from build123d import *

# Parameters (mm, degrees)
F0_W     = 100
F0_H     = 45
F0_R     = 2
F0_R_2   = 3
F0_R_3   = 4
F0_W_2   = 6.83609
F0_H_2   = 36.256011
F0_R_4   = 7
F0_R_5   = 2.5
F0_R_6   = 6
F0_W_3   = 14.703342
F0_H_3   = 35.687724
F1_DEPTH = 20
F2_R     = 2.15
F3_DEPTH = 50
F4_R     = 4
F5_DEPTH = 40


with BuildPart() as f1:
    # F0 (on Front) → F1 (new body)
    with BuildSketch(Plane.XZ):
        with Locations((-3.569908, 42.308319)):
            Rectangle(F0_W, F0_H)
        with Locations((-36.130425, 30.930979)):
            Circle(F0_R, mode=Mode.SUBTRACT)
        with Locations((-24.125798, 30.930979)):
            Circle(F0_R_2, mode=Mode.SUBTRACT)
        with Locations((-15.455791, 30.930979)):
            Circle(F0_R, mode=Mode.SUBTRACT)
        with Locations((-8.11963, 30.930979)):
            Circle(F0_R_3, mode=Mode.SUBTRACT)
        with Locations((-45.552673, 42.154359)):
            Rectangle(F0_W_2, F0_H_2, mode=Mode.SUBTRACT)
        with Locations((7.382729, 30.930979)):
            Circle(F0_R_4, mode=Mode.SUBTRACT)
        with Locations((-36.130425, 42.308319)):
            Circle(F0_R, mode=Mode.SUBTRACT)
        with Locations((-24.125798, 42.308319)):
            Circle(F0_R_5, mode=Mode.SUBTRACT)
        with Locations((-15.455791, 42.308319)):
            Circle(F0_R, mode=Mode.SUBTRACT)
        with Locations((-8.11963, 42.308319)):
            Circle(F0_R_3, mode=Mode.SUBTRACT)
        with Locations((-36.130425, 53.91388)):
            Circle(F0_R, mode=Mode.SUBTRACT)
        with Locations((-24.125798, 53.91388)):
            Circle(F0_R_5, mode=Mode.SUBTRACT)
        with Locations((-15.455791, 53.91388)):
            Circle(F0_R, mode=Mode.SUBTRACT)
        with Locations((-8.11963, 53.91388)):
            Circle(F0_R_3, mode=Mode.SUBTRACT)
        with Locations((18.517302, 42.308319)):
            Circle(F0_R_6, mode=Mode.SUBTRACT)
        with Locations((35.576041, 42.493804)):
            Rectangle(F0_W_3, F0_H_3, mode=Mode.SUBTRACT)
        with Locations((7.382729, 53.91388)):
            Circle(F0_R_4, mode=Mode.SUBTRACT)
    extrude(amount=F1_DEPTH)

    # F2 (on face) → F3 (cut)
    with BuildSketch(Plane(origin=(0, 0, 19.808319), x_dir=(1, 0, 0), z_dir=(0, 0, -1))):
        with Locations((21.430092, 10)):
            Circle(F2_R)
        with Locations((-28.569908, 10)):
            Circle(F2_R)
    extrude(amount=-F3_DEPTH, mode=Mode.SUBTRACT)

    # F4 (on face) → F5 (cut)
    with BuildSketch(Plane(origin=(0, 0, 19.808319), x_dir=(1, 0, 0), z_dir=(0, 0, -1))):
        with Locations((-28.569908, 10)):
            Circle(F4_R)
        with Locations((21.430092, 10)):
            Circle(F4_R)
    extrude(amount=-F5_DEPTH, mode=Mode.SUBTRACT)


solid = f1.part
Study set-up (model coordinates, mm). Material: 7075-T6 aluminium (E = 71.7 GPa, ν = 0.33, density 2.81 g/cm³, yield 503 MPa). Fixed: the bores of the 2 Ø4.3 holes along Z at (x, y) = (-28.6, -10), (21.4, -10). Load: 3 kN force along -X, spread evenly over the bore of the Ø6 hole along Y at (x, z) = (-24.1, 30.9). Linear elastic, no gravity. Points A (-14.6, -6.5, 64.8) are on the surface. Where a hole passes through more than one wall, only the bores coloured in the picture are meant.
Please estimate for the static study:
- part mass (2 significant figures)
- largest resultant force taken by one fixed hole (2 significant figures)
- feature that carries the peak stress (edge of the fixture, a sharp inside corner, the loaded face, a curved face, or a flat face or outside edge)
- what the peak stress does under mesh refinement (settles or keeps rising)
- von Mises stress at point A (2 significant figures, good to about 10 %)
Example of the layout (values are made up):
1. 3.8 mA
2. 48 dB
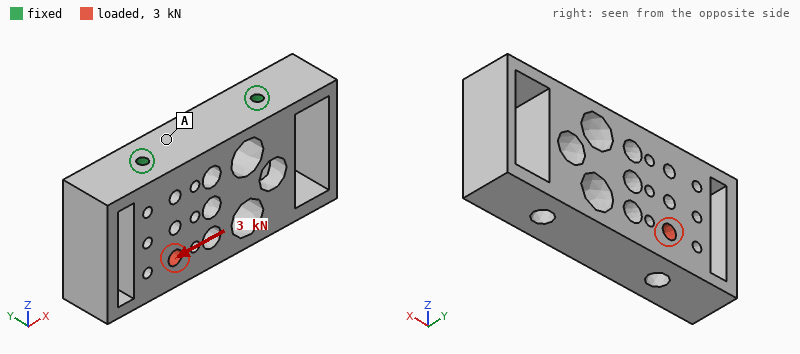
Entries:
1. 160 g
2. 2.4 kN
3. edge of the fixture
4. keeps rising
5. 7.4 MPa
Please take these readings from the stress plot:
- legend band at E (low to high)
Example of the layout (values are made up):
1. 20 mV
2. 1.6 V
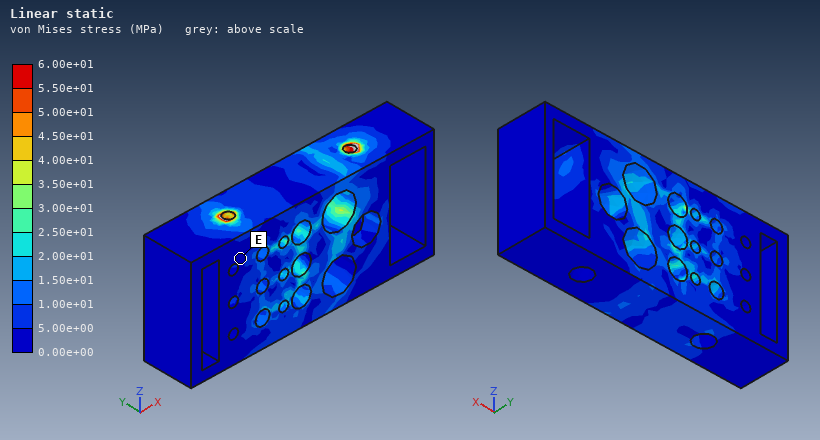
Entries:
1. 0.00e+00 to 5.00e+00 MPa
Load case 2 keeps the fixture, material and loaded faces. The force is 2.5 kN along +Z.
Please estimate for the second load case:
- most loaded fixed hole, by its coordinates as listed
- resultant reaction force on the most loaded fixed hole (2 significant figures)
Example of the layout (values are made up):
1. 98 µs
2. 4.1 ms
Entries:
1. (-28.6, -10)
2. 2.2 kN
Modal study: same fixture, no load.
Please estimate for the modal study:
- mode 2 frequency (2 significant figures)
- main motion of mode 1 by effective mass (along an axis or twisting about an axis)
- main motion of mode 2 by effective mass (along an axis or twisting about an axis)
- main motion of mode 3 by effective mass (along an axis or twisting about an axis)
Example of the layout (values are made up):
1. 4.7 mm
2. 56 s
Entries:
1. 4400 Hz
2. along Y
3. twisting about Z
4. along X
